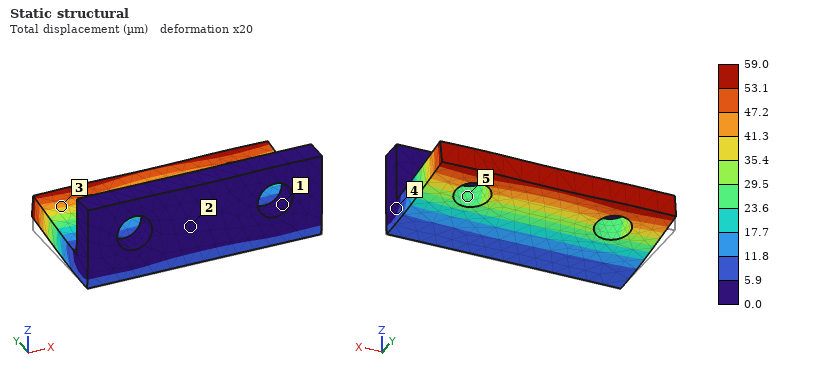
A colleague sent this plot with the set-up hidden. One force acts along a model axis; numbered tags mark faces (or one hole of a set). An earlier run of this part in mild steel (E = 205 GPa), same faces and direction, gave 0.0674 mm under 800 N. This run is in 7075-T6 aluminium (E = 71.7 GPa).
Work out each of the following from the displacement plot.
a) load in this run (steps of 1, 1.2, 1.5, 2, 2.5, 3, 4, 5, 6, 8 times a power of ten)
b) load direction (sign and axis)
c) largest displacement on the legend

250 N
+Z
59.0 µm
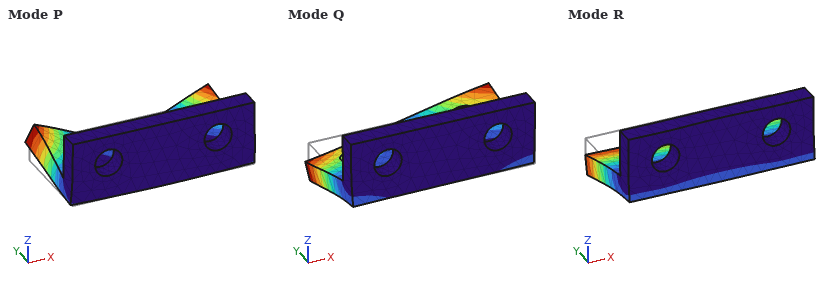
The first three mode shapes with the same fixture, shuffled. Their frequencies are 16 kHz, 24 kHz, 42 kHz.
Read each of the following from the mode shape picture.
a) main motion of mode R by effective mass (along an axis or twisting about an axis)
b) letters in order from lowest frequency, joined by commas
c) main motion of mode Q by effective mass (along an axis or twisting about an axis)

along Z
R, Q, P
twisting about Y
